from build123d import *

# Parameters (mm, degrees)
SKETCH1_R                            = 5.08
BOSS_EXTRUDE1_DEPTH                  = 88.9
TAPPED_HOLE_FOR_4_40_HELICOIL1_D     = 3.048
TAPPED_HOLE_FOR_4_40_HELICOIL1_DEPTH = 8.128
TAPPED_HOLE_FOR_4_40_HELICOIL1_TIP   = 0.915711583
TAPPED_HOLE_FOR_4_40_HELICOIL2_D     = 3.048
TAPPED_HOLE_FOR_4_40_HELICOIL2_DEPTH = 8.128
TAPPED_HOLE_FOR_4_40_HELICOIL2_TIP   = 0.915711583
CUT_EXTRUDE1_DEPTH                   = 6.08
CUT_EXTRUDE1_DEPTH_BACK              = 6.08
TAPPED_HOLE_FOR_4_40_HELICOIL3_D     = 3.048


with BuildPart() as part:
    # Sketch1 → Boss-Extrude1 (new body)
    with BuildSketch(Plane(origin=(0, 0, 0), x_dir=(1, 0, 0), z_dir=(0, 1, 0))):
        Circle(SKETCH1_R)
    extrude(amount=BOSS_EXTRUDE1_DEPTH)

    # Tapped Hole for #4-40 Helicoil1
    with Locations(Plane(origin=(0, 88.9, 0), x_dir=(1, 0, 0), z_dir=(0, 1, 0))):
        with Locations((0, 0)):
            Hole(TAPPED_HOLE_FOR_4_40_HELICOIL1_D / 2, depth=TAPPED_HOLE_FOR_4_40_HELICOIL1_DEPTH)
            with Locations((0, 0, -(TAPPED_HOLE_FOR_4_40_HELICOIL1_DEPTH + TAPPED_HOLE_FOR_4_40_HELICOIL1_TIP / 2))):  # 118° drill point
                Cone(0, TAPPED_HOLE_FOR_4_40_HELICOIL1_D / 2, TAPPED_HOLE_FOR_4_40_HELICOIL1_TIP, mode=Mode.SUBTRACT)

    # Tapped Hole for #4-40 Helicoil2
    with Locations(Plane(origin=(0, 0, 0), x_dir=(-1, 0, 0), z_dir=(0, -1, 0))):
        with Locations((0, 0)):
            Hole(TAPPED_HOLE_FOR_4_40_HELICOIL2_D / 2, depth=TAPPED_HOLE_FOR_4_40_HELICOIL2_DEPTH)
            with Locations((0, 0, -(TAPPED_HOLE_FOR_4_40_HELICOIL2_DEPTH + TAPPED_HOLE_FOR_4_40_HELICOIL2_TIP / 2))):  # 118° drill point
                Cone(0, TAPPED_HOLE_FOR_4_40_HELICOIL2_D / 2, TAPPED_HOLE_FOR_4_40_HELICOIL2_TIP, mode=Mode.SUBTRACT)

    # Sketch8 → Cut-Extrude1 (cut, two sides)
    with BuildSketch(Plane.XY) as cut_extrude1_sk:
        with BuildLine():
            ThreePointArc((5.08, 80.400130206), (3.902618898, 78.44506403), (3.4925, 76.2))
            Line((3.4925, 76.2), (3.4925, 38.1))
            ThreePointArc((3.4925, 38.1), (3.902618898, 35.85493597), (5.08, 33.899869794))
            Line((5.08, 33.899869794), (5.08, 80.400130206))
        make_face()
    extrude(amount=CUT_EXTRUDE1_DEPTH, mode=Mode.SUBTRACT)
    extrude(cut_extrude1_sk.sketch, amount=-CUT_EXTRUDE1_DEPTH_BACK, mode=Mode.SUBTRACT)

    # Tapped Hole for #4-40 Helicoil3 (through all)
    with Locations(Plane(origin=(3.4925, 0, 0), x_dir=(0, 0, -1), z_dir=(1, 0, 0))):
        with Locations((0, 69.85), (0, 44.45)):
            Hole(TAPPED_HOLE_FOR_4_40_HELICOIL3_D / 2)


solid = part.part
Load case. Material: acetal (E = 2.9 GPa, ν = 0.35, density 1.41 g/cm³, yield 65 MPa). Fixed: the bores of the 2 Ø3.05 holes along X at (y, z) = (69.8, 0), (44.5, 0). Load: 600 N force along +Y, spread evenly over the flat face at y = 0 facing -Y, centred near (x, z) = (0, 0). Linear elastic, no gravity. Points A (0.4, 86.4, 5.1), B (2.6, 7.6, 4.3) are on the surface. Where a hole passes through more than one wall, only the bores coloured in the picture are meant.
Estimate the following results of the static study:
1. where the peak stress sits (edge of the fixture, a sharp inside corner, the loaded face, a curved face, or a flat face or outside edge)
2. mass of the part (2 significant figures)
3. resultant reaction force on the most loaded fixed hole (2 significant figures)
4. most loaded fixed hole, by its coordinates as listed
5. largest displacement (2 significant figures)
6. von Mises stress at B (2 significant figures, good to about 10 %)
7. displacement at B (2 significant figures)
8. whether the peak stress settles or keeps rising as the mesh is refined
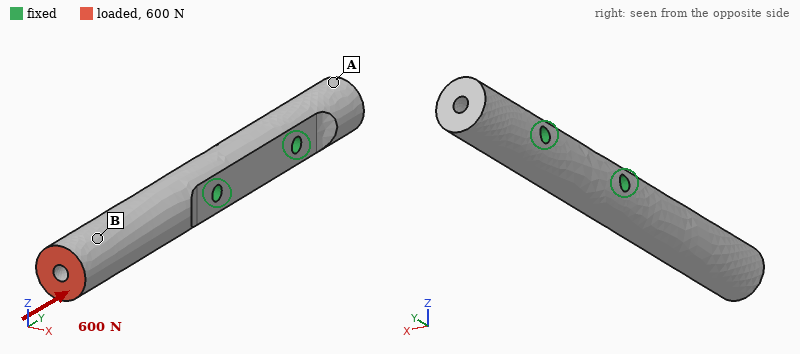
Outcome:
edge of the fixture
9.3 g
580 N
(44.5, 0)
0.17 mm
7.8 MPa
0.14 mm
keeps rising
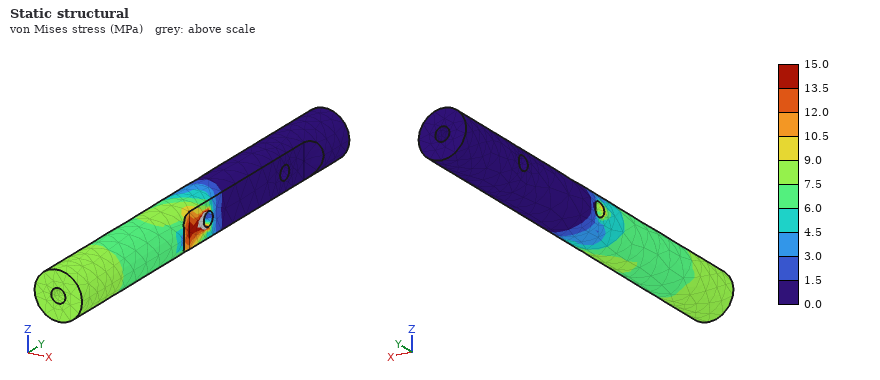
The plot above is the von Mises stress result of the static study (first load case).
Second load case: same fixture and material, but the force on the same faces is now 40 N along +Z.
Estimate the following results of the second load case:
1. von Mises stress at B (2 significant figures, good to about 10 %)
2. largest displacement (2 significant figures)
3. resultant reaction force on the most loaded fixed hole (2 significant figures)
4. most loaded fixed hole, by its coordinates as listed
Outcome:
2.7 MPa
0.97 mm
70 N
(44.5, 0)
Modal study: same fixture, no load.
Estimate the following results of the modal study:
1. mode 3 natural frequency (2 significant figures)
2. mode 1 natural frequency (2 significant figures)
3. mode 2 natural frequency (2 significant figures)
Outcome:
4200 Hz
910 Hz
940 Hz
